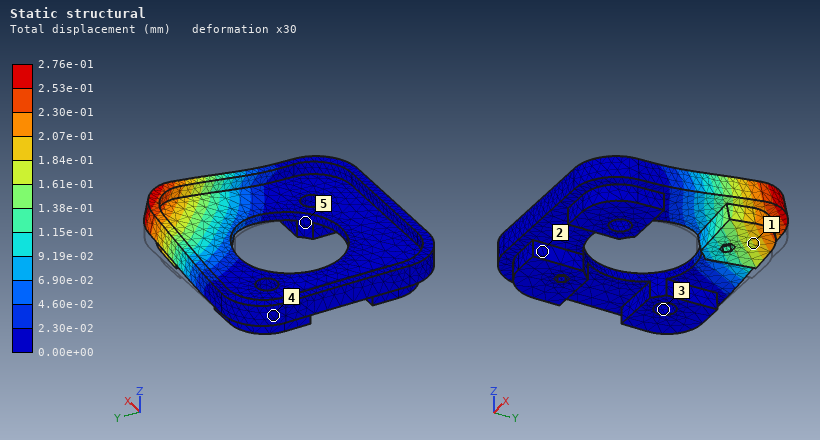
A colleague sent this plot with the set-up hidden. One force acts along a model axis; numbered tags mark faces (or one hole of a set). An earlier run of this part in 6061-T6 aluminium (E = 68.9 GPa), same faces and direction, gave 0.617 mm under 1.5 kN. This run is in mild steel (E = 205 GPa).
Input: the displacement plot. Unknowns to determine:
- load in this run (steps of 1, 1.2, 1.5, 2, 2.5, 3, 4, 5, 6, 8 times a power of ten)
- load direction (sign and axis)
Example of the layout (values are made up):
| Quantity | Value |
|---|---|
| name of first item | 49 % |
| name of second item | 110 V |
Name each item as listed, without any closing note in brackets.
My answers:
| Quantity | Value |
|---|---|
| load in this run | 2 kN |
| load direction | +Z |
